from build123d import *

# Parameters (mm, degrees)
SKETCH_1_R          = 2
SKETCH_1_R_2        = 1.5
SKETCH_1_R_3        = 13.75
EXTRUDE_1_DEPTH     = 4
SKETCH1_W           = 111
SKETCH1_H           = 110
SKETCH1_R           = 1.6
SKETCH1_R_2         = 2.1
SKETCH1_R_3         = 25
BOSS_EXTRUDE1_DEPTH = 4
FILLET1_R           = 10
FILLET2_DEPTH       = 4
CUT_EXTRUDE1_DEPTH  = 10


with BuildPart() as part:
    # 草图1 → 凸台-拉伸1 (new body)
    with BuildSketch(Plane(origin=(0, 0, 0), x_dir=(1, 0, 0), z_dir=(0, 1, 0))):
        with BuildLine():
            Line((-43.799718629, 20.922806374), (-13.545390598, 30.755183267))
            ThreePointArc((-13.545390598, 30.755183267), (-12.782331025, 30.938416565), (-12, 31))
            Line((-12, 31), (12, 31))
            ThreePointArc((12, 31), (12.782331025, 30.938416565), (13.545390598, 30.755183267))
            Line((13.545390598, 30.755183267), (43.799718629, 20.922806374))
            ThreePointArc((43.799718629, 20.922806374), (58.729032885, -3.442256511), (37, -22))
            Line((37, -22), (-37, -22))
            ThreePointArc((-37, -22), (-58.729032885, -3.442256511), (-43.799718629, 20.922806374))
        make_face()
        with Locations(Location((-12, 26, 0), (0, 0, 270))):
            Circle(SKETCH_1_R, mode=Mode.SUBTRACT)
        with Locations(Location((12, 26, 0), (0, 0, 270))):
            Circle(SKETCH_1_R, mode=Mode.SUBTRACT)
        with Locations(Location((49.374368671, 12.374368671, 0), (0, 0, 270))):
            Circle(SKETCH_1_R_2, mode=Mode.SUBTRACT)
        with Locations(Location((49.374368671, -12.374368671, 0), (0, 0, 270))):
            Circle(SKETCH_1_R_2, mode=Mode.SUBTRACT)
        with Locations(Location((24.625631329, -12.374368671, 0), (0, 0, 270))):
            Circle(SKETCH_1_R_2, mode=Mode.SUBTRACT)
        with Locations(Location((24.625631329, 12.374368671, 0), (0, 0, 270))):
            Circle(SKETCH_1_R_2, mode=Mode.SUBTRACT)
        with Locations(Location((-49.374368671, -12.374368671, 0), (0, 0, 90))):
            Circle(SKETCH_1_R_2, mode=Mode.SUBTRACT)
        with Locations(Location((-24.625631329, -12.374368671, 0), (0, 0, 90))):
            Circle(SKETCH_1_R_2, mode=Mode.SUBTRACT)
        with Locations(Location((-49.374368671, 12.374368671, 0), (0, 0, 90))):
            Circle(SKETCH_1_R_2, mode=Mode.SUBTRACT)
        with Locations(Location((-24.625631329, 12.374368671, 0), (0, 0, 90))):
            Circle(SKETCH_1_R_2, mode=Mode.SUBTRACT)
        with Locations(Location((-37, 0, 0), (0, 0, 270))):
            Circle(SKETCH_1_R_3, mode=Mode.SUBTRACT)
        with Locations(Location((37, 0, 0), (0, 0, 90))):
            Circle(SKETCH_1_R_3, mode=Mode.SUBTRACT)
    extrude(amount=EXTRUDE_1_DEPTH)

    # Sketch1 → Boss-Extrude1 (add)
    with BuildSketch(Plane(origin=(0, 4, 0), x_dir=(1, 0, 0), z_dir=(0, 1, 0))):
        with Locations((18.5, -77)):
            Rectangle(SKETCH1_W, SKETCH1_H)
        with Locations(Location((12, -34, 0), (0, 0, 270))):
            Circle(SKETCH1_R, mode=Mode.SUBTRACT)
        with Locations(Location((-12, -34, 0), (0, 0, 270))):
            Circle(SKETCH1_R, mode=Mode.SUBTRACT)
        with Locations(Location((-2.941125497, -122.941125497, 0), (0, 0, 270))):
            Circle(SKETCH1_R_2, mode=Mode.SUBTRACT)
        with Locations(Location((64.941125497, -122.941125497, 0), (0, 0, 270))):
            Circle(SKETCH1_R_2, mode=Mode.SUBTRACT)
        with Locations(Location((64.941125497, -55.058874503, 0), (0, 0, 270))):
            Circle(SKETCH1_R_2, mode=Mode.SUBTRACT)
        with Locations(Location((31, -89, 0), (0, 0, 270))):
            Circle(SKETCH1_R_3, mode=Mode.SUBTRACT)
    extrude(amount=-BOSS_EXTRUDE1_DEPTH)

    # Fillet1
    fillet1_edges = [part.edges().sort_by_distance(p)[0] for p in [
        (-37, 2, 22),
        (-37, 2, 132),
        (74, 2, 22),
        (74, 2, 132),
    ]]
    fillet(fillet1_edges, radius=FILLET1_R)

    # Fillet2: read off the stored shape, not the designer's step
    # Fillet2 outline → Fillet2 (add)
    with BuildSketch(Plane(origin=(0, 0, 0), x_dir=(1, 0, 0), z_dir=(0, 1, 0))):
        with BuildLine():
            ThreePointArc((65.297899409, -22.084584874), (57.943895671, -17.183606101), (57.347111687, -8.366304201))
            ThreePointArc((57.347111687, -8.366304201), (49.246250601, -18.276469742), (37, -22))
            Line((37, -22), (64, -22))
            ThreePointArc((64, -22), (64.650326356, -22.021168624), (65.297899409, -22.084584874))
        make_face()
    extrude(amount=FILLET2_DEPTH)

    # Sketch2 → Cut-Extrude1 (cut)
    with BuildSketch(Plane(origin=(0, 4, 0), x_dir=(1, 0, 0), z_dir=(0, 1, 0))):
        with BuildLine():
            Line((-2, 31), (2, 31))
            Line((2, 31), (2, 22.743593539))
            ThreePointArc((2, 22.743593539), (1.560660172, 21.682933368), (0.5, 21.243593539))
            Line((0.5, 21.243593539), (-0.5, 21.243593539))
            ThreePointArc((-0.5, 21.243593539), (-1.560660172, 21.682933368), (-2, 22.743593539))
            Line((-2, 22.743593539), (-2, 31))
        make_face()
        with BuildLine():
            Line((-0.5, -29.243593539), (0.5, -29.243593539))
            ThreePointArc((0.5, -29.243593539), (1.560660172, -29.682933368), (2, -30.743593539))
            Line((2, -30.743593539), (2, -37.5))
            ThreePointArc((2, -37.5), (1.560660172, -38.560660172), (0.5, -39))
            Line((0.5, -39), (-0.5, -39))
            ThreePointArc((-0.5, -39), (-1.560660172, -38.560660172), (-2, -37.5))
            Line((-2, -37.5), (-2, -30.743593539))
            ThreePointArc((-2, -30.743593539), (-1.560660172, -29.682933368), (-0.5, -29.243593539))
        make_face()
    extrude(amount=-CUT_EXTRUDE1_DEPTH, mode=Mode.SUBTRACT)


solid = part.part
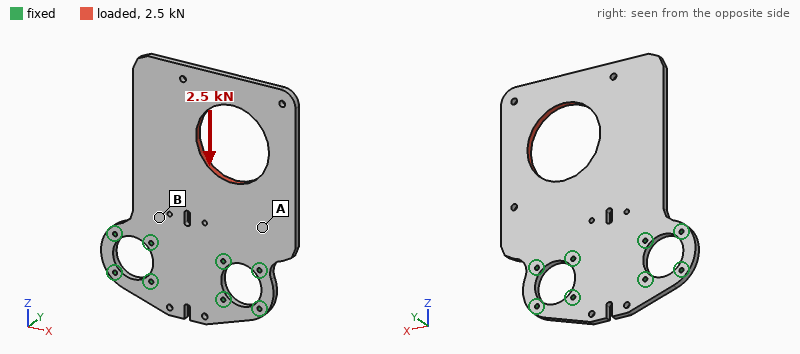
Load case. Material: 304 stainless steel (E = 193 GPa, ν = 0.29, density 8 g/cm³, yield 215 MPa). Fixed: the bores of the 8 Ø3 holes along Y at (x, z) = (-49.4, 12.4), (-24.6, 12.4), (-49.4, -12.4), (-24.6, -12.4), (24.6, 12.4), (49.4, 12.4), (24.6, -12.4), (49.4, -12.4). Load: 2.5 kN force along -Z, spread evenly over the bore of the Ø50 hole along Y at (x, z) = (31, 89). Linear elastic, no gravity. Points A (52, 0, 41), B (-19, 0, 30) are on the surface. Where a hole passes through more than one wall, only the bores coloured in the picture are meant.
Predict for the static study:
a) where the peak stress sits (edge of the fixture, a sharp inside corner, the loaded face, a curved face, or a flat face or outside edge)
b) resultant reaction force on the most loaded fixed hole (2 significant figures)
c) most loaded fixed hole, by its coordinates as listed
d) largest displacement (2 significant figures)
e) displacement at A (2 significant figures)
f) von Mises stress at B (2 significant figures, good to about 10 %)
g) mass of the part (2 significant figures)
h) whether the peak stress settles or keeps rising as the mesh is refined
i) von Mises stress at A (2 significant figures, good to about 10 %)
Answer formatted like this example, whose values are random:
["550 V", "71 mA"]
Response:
["edge of the fixture", "1.2 kN", "(49.4, 12.4)", "11 µm", "3.0 µm", "3.2 MPa", "450 g", "keeps rising", "11 MPa"]
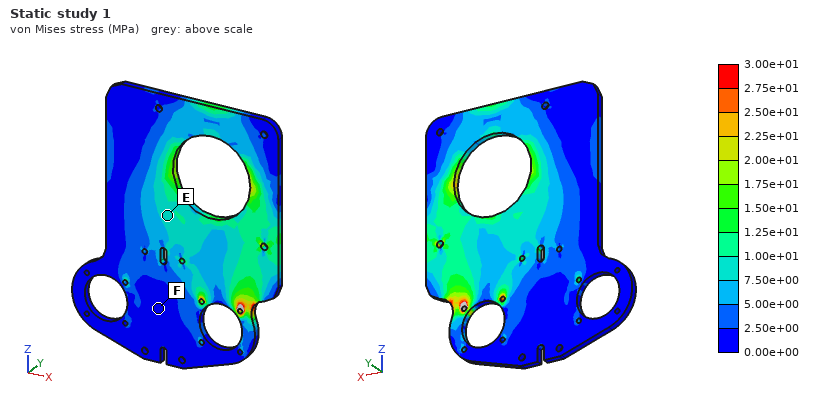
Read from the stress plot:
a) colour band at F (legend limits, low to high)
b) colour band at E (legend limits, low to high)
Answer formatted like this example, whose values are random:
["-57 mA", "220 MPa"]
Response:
["0.00e+00 to 2.50e+00 MPa", "7.50e+00 to 1.00e+01 MPa"]
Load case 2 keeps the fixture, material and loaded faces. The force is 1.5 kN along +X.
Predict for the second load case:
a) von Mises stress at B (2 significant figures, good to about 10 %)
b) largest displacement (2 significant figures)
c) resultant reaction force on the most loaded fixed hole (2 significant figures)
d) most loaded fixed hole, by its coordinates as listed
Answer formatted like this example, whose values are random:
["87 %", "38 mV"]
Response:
["11 MPa", "20 µm", "1.2 kN", "(49.4, 12.4)"]
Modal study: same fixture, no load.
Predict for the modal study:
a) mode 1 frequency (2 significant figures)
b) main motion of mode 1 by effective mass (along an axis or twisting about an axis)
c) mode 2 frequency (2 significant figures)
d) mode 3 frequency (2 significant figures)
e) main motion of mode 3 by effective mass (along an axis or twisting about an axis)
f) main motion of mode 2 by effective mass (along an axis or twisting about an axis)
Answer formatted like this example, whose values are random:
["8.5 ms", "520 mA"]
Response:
["220 Hz", "along Y", "520 Hz", "1200 Hz", "along Y", "twisting about Z"]
